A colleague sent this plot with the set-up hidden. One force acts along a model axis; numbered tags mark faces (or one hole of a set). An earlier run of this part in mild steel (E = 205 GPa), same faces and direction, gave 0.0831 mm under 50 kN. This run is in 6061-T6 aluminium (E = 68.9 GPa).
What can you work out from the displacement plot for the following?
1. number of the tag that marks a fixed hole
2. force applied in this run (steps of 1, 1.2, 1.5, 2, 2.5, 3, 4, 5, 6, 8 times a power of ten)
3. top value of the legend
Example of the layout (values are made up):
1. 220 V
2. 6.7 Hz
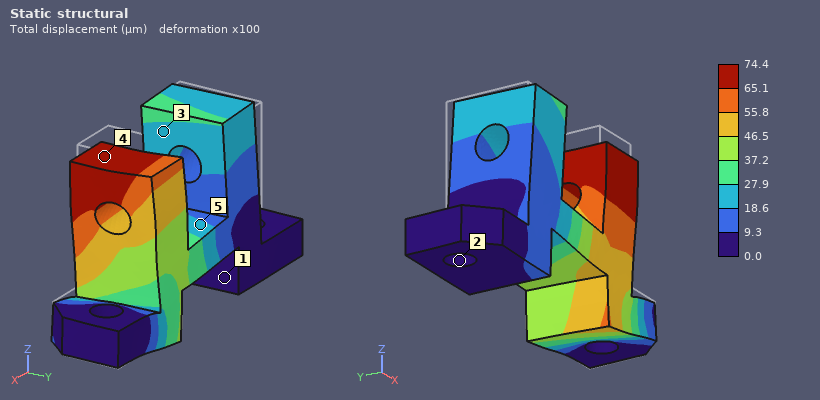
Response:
1. 2
2. 15 kN
3. 74.4 µm
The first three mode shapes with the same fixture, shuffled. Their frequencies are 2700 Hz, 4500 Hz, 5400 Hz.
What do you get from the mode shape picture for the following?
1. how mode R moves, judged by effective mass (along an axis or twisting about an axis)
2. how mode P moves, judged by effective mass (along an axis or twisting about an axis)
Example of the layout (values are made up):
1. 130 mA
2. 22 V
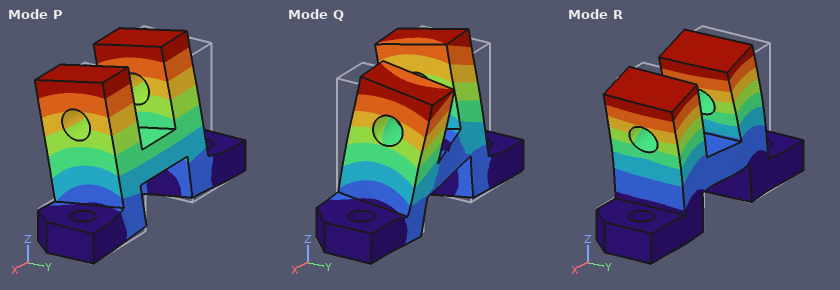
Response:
1. along X
2. along Y
